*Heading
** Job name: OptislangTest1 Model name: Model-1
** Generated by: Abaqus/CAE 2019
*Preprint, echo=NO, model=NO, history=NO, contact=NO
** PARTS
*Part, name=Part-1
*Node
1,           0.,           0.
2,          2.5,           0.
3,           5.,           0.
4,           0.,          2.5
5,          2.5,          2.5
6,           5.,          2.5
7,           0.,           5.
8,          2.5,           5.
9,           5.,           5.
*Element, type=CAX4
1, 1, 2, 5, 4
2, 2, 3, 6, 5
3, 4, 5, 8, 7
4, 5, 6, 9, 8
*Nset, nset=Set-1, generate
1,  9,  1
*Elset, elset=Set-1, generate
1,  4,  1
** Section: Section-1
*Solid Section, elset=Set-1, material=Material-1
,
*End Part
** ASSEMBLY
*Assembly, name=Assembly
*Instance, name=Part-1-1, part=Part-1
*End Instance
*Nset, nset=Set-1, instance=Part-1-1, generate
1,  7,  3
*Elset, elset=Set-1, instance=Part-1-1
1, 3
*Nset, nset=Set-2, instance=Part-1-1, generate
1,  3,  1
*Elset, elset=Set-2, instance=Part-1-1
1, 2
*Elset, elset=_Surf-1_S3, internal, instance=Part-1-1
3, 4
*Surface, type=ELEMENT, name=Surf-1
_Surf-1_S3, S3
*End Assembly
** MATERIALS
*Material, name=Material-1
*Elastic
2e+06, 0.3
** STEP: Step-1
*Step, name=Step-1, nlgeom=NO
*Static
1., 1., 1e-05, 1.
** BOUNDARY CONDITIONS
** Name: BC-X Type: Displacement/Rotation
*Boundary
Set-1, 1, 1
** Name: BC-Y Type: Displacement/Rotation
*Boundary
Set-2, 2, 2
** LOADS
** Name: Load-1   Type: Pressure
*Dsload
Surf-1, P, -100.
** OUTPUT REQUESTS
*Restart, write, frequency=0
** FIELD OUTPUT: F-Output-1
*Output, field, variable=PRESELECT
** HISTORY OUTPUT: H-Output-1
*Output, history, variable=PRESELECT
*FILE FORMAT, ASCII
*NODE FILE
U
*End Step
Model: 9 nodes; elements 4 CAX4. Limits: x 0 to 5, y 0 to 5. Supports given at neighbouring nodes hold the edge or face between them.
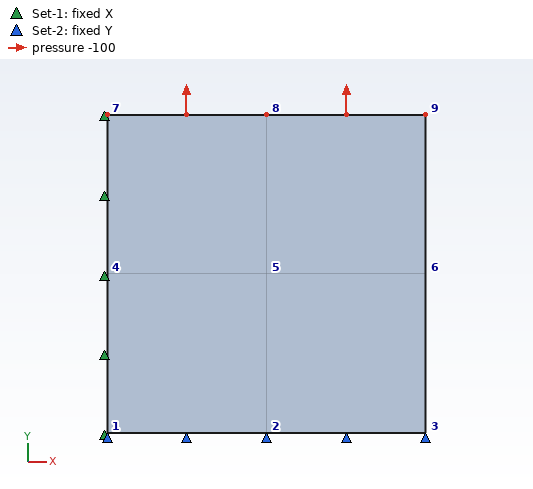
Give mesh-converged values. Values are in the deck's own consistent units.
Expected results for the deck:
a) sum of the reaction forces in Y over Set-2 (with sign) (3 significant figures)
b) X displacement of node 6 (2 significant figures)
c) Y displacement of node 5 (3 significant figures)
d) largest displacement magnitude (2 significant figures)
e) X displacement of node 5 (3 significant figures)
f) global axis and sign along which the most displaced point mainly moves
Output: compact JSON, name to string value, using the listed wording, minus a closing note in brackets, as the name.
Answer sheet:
{"sum of the reaction forces in Y over Set-2 (with sign)": "-7850", "X displacement of node 6": "-7.5e-05", "Y displacement of node 5": "1.25e-04", "largest displacement magnitude": "2.6e-04", "X displacement of node 5": "-3.75e-05", "global axis and sign along which the most displaced point mainly moves": "+Y"}
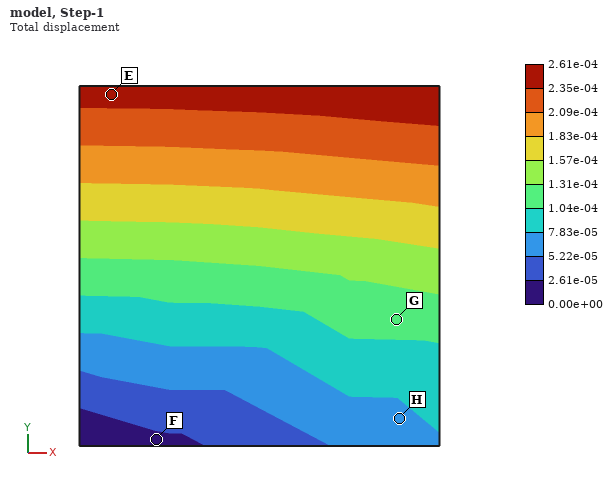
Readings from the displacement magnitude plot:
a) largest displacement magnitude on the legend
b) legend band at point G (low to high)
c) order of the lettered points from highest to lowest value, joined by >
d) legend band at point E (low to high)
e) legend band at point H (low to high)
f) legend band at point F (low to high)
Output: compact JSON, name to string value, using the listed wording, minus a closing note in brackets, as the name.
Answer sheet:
{"largest displacement magnitude on the legend": "2.61e-04", "legend band at point G": "1.04e-04 to 1.31e-04", "order of the lettered points from highest to lowest value, joined by >": "E > G > H > F", "legend band at point E": "2.35e-04 to 2.61e-04", "legend band at point H": "5.22e-05 to 7.83e-05", "legend band at point F": "0.00e+00 to 2.61e-05"}
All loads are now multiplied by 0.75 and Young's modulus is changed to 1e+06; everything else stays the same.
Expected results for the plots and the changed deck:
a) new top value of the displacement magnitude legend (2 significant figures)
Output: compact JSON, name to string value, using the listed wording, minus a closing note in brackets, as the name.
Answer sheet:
{"new top value of the displacement magnitude legend": "3.9e-04"}
